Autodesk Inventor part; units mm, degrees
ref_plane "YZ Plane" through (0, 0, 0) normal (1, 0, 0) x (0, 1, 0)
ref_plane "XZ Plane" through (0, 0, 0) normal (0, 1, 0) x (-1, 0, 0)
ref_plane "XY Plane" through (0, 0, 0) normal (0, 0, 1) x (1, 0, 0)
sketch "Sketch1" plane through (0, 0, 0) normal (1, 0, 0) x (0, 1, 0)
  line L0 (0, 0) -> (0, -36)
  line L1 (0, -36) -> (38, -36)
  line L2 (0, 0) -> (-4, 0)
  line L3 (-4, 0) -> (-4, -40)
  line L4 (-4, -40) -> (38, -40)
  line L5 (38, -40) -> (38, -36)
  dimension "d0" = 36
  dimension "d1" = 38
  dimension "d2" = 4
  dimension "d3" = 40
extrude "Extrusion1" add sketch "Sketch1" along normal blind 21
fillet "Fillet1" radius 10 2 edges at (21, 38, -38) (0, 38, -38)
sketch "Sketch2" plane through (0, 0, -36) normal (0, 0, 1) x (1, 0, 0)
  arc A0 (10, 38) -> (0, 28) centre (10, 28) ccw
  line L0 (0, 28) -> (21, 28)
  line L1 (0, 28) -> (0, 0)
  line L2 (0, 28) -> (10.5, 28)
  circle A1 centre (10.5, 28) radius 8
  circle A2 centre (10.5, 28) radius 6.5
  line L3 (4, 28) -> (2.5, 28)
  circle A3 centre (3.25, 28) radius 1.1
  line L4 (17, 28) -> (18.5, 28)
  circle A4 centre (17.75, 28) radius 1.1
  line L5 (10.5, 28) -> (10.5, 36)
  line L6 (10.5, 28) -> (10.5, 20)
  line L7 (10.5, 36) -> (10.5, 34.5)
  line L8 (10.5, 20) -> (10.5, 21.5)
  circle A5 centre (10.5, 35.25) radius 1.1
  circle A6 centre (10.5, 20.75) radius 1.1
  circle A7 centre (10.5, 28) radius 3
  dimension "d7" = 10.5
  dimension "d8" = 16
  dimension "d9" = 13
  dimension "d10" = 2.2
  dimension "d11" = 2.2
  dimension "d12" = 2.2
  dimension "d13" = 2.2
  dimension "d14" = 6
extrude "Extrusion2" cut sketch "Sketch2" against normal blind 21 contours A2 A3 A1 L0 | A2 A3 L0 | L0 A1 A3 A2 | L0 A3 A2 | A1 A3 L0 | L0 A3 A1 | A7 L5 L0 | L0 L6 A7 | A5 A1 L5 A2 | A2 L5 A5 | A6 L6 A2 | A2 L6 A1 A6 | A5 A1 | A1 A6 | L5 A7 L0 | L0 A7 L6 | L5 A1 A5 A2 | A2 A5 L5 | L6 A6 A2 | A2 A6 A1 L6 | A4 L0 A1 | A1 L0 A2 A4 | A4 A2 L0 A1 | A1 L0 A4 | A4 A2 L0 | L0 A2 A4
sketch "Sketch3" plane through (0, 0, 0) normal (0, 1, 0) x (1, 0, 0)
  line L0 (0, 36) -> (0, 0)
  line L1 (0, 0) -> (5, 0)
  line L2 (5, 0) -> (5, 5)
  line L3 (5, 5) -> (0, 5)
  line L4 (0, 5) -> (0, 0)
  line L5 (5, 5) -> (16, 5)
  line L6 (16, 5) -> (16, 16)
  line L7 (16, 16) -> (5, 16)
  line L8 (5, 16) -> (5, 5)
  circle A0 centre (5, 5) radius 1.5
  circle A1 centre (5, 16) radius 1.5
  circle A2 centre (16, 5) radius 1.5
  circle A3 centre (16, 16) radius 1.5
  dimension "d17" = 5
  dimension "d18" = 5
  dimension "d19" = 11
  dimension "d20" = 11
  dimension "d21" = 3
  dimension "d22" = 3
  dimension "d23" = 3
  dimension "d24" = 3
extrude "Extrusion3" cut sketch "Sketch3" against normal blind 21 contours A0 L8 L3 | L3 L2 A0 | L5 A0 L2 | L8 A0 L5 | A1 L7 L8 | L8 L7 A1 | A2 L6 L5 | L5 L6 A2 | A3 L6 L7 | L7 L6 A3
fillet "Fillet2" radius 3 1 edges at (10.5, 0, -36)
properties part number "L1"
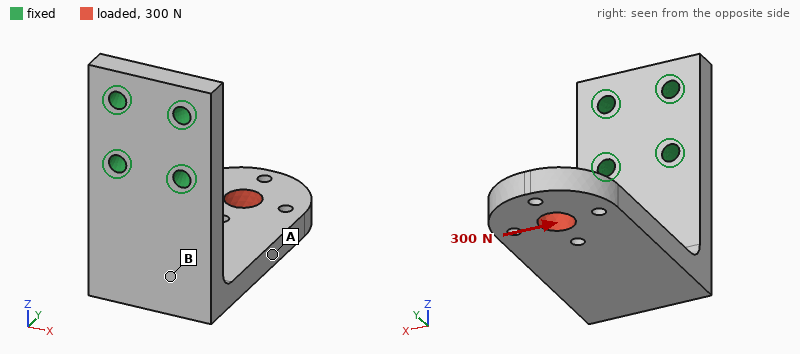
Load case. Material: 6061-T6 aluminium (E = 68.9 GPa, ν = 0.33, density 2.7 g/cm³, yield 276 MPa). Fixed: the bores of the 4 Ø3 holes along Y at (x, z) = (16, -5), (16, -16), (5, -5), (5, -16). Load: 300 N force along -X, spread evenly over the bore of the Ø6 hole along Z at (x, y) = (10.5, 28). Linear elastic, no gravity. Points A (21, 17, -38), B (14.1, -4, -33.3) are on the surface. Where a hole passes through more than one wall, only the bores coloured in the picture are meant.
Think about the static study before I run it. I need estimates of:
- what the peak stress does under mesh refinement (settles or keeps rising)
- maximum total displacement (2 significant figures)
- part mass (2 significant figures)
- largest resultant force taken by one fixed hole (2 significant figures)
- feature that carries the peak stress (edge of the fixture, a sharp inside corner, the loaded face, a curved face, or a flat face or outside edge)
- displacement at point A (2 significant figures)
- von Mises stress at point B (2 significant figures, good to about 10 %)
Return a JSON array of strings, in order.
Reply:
["keeps rising", "0.49 mm", "17 g", "790 N", "edge of the fixture", "0.26 mm", "91 MPa"]
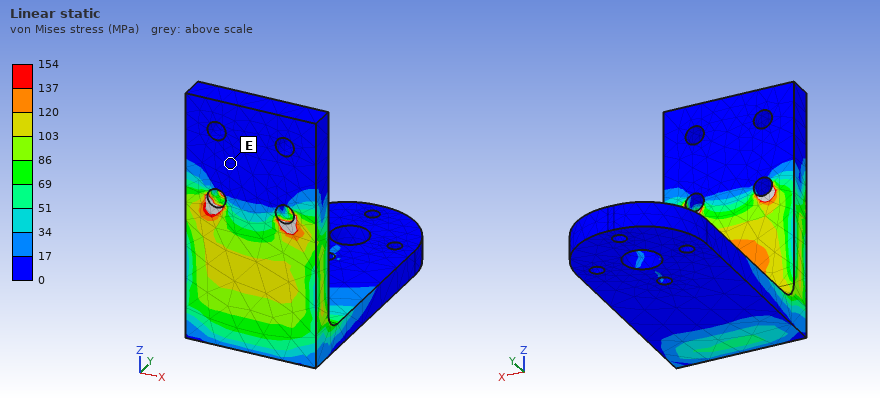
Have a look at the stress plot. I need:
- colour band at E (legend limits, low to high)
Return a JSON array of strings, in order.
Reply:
["0 to 17 MPa"]
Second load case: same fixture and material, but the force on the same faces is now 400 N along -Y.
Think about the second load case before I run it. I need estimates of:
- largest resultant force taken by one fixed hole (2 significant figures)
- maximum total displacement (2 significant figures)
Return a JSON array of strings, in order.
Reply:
["280 N", "0.51 mm"]
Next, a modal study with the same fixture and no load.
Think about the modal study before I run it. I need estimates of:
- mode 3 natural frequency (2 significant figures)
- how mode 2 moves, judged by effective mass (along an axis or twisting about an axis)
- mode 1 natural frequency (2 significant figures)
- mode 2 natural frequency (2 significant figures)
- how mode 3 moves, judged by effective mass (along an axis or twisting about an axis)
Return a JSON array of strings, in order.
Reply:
["4100 Hz", "along X", "1300 Hz", "2100 Hz", "along Y"]
